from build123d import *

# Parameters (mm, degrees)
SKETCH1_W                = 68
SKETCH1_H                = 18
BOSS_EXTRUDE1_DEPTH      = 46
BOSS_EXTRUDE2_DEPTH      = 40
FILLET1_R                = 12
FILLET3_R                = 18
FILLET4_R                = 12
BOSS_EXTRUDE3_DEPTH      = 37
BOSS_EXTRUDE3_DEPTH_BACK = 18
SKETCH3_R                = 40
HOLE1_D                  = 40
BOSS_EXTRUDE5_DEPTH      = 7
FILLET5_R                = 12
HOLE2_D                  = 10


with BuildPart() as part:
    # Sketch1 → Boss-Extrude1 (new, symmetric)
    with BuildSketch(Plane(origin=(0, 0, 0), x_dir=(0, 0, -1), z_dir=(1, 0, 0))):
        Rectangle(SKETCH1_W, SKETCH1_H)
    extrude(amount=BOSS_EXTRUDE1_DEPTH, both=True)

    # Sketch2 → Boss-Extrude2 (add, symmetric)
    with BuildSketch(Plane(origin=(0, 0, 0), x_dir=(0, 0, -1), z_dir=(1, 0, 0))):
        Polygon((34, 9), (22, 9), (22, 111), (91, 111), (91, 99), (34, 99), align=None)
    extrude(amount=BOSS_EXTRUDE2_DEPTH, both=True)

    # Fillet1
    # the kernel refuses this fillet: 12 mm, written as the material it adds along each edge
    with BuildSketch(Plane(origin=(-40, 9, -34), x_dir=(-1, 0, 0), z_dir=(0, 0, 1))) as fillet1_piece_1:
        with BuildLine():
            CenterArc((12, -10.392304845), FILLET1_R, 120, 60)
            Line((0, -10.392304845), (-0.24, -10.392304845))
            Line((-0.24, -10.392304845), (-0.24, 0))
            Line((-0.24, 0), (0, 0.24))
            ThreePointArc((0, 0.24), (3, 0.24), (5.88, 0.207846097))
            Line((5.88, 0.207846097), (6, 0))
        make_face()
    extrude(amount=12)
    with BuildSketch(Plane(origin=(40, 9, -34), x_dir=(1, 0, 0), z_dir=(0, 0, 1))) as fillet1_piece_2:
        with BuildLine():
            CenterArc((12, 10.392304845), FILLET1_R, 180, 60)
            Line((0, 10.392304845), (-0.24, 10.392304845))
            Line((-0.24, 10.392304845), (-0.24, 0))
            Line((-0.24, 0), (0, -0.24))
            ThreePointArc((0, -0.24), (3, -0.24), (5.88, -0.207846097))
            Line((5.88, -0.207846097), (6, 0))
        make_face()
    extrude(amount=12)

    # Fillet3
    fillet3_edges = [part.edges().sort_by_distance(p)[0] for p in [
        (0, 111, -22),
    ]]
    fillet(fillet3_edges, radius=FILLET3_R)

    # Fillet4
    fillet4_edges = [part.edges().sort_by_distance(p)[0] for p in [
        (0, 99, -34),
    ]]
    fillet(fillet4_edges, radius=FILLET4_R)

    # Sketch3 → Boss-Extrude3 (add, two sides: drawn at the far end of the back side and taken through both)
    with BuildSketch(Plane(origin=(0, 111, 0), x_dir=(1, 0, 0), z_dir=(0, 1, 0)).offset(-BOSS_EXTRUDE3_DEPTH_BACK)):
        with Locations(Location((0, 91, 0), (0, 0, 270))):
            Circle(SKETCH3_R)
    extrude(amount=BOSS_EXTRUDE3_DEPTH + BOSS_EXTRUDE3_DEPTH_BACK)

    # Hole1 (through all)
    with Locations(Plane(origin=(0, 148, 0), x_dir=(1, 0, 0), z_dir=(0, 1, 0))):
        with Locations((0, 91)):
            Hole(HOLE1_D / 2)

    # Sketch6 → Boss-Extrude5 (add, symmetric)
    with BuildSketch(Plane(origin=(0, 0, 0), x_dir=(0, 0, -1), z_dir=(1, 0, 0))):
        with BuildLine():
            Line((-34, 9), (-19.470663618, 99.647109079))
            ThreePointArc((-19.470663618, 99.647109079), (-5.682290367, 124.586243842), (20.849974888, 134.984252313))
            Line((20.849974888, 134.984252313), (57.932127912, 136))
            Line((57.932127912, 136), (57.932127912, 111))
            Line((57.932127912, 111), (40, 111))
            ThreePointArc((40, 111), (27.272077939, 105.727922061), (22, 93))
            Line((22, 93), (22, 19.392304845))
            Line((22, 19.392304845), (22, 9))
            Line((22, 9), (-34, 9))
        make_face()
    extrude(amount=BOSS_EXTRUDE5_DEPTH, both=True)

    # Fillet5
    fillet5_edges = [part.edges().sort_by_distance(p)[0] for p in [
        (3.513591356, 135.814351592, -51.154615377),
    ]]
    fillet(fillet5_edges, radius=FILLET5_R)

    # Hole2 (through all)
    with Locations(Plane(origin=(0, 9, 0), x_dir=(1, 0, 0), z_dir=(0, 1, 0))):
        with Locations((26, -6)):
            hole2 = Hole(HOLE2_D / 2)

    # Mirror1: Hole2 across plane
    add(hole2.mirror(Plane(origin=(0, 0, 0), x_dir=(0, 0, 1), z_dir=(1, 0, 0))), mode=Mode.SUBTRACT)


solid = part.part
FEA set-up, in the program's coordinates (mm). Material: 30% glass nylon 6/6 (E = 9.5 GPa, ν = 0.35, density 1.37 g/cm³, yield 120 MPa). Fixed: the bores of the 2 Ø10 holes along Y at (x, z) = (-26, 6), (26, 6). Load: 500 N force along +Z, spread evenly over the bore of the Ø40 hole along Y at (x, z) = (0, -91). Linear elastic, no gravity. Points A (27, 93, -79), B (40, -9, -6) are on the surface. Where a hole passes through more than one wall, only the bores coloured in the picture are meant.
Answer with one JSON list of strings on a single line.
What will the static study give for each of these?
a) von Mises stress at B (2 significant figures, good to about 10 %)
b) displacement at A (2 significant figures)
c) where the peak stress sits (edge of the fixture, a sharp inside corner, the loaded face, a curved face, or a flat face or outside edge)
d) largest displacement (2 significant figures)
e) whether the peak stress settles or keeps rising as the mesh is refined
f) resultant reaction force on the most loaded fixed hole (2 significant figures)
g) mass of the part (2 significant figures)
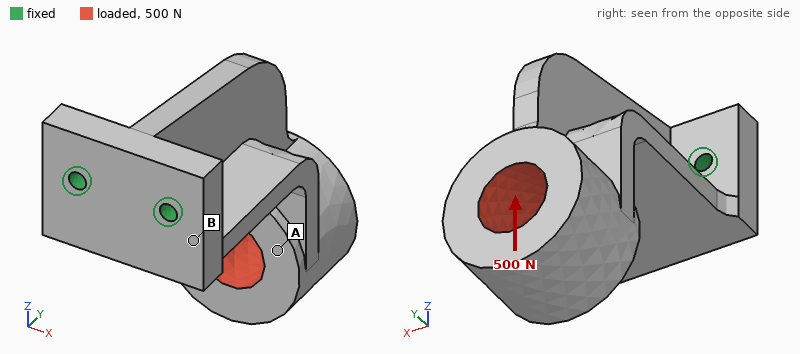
["3.8 MPa", "0.27 mm", "edge of the fixture", "0.47 mm", "keeps rising", "250 N", "720 g"]
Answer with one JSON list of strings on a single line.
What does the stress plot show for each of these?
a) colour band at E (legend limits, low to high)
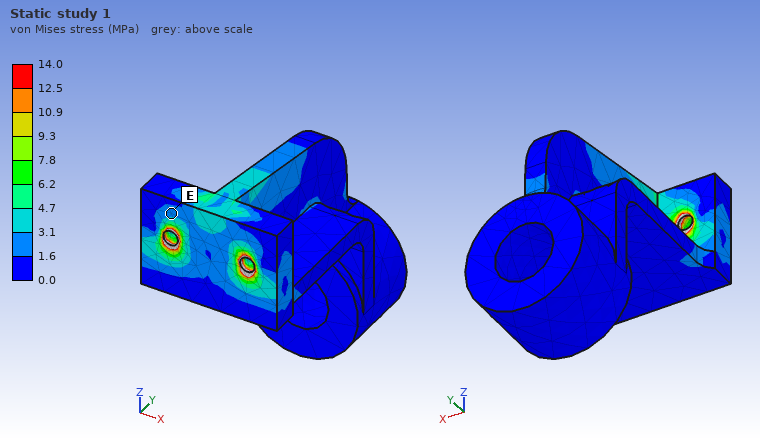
["1.6 to 3.1 MPa"]
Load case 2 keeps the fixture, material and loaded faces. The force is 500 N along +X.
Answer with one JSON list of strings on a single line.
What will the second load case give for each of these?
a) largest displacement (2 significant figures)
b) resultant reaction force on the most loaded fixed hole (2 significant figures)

["1.0 mm", "1.3 kN"]
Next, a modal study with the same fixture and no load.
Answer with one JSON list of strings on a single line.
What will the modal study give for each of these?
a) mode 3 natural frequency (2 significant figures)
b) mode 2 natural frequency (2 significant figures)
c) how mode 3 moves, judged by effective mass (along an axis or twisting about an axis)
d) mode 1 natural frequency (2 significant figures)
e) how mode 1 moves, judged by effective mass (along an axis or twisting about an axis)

["600 Hz", "270 Hz", "along X", "230 Hz", "along X"]
